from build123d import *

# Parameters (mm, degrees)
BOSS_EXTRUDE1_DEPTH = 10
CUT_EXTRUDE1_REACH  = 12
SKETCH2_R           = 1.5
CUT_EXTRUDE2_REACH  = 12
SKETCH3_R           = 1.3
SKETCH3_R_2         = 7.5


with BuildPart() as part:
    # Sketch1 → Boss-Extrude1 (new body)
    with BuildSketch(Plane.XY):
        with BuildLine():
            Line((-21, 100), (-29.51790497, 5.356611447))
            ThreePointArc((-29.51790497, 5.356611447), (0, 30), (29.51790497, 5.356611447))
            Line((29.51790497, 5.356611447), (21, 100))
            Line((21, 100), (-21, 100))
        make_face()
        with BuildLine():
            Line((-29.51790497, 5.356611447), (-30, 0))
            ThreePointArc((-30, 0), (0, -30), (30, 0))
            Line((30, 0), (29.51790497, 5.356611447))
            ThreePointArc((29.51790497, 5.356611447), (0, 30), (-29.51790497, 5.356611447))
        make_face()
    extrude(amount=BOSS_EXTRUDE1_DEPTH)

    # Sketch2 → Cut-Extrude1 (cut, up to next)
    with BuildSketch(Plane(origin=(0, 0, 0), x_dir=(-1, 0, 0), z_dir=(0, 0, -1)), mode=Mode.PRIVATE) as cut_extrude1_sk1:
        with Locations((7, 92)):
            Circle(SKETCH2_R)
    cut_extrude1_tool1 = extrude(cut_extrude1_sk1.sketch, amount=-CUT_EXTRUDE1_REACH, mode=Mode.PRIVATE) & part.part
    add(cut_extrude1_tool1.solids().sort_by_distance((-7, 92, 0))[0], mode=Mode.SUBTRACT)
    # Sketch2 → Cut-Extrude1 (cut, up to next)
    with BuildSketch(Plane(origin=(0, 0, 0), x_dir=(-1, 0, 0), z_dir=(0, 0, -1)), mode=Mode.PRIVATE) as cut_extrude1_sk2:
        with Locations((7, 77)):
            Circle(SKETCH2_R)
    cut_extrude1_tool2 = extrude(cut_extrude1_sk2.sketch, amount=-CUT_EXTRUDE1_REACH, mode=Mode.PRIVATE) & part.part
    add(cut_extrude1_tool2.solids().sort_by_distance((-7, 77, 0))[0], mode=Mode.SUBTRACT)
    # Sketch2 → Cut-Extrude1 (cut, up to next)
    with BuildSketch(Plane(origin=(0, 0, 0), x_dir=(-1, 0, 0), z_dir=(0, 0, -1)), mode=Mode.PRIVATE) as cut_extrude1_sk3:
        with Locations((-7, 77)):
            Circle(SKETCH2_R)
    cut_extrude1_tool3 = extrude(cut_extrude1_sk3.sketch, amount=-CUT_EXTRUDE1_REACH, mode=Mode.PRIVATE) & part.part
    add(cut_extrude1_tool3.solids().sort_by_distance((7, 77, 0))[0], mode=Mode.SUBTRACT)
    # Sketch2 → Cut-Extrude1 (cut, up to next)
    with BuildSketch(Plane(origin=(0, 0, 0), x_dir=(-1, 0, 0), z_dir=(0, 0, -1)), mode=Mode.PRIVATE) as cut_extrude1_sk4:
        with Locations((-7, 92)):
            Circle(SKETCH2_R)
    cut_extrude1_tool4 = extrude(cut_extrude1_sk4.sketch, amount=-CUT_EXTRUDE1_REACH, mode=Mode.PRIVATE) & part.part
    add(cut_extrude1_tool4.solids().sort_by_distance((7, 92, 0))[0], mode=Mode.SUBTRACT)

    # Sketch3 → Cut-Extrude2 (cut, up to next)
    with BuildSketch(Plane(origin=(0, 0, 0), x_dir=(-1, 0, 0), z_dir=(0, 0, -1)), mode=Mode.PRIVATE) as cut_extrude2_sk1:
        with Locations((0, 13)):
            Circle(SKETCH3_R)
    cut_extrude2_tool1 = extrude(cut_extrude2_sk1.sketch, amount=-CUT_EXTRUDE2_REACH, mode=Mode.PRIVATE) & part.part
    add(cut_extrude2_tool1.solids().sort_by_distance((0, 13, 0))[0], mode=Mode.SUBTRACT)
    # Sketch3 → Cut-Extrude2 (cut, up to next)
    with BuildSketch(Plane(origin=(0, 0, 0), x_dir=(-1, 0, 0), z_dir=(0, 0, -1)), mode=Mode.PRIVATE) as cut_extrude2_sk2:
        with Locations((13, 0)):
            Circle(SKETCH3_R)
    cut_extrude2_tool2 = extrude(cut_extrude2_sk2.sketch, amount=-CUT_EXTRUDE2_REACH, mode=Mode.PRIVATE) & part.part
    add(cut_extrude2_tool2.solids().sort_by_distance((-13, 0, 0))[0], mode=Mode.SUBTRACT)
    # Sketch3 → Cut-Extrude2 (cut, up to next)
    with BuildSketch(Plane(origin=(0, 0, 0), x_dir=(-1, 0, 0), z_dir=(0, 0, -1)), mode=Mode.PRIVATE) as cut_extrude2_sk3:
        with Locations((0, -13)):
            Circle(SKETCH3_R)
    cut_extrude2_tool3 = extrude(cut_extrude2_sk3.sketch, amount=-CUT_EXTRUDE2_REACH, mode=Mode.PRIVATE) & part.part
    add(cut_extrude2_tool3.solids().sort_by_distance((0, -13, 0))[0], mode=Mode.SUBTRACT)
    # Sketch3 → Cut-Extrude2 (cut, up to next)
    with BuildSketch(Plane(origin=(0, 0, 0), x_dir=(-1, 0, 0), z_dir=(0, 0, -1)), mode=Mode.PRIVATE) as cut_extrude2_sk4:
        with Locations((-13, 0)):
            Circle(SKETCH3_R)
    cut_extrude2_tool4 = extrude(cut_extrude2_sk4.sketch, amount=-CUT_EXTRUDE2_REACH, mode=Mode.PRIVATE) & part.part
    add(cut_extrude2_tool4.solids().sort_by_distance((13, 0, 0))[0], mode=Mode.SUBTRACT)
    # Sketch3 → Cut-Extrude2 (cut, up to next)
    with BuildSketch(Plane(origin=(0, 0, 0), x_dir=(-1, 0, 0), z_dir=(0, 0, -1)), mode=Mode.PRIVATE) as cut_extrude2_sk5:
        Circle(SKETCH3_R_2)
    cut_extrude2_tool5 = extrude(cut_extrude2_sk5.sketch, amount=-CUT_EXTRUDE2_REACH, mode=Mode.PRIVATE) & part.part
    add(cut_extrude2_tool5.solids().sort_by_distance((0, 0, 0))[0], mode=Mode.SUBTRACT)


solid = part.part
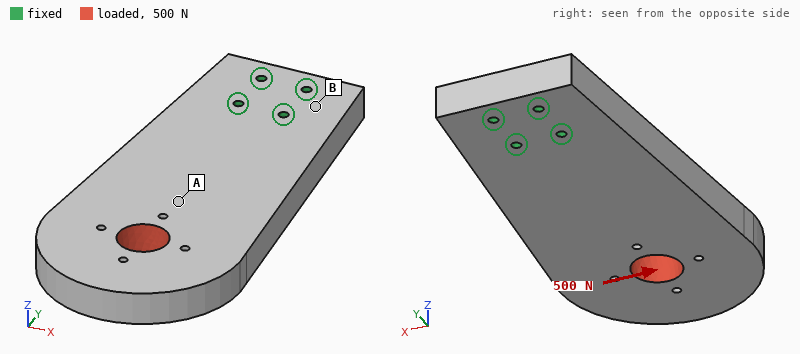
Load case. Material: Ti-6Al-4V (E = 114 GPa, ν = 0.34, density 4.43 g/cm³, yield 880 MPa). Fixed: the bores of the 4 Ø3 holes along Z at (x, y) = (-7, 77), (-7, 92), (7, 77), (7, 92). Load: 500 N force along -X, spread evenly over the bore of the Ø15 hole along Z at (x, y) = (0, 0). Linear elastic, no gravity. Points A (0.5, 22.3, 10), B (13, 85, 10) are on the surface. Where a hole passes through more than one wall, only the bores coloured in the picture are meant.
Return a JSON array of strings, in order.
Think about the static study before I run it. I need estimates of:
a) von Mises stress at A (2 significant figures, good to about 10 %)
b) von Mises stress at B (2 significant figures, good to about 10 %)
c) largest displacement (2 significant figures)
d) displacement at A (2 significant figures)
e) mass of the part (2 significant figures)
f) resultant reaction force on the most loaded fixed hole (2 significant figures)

["3.0 MPa", "7.6 MPa", "21 µm", "10 µm", "280 g", "1.3 kN"]
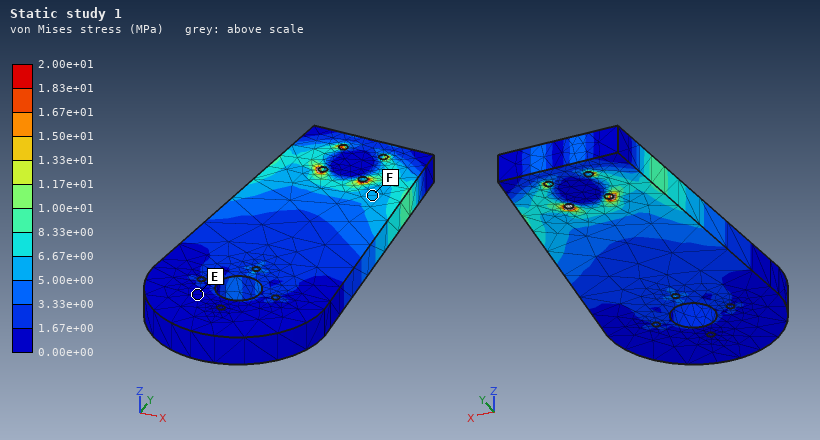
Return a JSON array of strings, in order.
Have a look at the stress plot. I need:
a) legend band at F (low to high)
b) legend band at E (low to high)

["5.00e+00 to 6.67e+00 MPa", "0.00e+00 to 1.67e+00 MPa"]
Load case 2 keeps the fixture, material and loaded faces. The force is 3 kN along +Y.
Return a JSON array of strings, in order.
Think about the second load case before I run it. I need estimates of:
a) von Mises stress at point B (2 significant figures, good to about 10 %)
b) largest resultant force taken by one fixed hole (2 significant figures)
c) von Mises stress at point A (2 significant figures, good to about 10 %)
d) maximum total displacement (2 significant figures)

["4.4 MPa", "1.2 kN", "6.5 MPa", "5.8 µm"]
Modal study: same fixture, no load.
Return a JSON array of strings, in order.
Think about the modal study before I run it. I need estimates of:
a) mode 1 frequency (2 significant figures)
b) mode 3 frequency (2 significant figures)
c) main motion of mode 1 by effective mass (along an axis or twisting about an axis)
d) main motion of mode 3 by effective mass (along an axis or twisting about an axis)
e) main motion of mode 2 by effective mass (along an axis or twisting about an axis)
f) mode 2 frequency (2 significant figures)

["730 Hz", "2600 Hz", "along Z", "twisting about Y", "along X", "2400 Hz"]
